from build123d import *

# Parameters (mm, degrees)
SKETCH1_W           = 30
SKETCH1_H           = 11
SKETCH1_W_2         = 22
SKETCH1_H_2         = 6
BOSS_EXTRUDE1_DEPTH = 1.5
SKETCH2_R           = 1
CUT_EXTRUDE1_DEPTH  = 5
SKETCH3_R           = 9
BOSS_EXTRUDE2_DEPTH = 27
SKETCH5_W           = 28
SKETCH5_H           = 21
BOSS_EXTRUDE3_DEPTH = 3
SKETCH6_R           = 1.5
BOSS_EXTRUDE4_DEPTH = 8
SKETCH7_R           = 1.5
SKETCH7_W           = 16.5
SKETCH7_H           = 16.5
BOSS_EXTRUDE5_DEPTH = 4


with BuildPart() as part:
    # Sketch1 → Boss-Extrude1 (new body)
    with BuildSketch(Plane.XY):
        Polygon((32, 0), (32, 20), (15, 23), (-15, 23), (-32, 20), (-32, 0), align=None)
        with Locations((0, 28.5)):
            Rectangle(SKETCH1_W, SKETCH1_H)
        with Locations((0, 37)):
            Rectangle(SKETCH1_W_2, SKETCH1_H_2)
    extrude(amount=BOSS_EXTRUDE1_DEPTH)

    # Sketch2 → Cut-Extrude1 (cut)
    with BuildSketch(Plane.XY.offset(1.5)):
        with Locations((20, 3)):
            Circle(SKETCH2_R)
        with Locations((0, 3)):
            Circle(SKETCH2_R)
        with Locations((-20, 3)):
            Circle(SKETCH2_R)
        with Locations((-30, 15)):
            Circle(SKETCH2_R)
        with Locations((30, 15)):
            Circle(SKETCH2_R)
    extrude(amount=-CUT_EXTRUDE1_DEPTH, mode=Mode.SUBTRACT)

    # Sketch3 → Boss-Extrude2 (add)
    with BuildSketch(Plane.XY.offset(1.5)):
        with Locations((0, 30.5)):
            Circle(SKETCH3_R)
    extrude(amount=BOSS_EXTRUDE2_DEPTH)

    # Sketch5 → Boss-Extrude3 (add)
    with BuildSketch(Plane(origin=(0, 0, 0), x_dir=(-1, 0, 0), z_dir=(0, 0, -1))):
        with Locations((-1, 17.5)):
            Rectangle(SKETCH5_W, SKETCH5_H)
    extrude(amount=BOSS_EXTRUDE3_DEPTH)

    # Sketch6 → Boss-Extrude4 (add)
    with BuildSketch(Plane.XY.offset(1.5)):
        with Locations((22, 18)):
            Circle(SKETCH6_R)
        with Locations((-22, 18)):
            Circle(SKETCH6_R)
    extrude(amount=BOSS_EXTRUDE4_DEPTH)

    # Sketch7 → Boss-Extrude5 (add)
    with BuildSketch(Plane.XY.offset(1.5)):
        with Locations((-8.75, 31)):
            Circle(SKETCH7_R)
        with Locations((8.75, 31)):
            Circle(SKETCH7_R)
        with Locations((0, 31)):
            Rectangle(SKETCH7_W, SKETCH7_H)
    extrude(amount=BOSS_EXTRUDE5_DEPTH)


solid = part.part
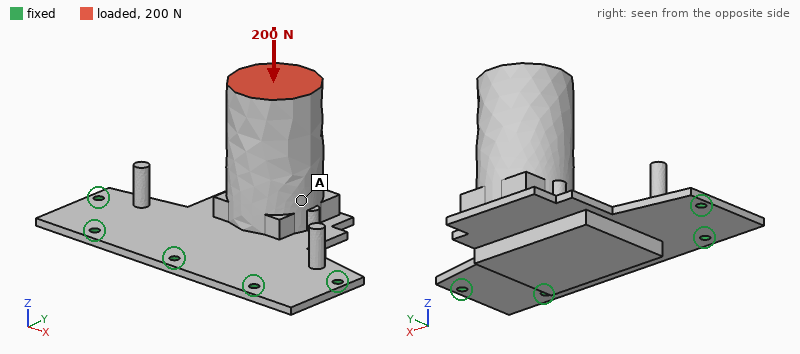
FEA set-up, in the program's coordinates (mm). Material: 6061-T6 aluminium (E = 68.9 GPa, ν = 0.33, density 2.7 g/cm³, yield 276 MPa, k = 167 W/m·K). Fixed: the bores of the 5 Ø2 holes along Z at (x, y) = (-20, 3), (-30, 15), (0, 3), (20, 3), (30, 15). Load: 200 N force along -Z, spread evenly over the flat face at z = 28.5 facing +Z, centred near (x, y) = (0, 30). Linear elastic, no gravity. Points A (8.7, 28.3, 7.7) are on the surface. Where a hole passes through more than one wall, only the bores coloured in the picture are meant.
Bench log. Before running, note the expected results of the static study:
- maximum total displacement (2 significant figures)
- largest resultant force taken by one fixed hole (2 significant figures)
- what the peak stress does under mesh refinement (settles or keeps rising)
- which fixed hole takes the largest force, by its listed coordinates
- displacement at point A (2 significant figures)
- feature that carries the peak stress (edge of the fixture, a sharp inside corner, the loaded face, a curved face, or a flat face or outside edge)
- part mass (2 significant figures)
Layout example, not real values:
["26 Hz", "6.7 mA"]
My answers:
["0.81 mm", "180 N", "keeps rising", "(30, 15)", "0.43 mm", "edge of the fixture", "32 g"]
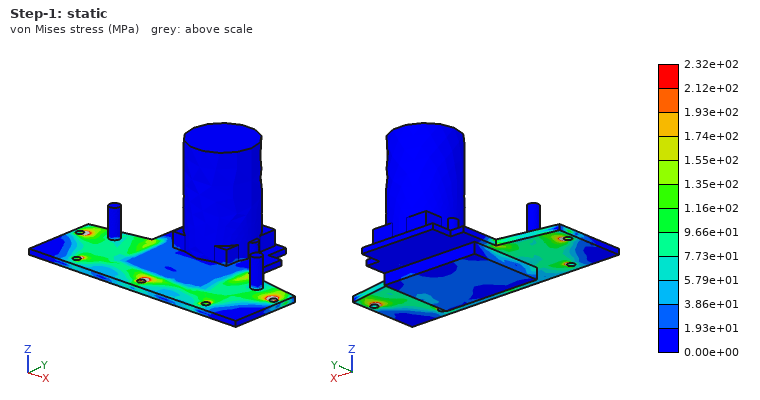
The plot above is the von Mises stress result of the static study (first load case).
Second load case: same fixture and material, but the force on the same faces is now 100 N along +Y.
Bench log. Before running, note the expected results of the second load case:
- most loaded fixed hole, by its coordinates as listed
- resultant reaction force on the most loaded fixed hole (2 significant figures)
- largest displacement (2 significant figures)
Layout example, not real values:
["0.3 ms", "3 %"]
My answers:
["(30, 15)", "110 N", "0.50 mm"]
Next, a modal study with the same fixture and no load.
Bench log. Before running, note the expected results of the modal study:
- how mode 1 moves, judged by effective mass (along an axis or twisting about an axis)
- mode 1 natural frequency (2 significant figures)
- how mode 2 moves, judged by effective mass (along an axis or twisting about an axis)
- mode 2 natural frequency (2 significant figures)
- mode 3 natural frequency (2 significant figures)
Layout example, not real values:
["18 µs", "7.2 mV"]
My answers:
["along Z", "590 Hz", "along X", "2000 Hz", "3600 Hz"]
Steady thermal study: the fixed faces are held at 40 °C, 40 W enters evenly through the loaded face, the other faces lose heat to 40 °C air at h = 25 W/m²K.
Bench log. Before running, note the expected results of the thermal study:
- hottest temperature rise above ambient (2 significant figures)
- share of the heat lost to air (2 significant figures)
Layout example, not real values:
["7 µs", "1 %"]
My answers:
["77 K", "13 %"]
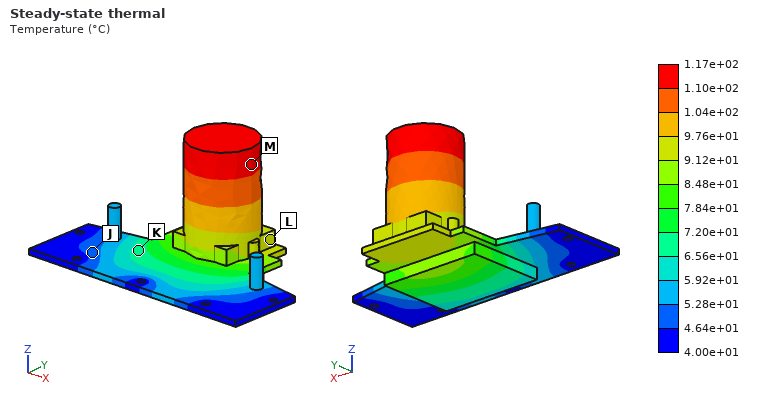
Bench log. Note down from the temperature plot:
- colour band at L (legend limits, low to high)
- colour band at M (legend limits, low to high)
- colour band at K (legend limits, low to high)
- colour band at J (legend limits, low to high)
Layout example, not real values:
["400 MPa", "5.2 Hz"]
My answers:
["9.12e+01 to 9.76e+01 °C", "1.10e+02 to 1.17e+02 °C", "6.56e+01 to 7.20e+01 °C", "4.64e+01 to 5.28e+01 °C"]
